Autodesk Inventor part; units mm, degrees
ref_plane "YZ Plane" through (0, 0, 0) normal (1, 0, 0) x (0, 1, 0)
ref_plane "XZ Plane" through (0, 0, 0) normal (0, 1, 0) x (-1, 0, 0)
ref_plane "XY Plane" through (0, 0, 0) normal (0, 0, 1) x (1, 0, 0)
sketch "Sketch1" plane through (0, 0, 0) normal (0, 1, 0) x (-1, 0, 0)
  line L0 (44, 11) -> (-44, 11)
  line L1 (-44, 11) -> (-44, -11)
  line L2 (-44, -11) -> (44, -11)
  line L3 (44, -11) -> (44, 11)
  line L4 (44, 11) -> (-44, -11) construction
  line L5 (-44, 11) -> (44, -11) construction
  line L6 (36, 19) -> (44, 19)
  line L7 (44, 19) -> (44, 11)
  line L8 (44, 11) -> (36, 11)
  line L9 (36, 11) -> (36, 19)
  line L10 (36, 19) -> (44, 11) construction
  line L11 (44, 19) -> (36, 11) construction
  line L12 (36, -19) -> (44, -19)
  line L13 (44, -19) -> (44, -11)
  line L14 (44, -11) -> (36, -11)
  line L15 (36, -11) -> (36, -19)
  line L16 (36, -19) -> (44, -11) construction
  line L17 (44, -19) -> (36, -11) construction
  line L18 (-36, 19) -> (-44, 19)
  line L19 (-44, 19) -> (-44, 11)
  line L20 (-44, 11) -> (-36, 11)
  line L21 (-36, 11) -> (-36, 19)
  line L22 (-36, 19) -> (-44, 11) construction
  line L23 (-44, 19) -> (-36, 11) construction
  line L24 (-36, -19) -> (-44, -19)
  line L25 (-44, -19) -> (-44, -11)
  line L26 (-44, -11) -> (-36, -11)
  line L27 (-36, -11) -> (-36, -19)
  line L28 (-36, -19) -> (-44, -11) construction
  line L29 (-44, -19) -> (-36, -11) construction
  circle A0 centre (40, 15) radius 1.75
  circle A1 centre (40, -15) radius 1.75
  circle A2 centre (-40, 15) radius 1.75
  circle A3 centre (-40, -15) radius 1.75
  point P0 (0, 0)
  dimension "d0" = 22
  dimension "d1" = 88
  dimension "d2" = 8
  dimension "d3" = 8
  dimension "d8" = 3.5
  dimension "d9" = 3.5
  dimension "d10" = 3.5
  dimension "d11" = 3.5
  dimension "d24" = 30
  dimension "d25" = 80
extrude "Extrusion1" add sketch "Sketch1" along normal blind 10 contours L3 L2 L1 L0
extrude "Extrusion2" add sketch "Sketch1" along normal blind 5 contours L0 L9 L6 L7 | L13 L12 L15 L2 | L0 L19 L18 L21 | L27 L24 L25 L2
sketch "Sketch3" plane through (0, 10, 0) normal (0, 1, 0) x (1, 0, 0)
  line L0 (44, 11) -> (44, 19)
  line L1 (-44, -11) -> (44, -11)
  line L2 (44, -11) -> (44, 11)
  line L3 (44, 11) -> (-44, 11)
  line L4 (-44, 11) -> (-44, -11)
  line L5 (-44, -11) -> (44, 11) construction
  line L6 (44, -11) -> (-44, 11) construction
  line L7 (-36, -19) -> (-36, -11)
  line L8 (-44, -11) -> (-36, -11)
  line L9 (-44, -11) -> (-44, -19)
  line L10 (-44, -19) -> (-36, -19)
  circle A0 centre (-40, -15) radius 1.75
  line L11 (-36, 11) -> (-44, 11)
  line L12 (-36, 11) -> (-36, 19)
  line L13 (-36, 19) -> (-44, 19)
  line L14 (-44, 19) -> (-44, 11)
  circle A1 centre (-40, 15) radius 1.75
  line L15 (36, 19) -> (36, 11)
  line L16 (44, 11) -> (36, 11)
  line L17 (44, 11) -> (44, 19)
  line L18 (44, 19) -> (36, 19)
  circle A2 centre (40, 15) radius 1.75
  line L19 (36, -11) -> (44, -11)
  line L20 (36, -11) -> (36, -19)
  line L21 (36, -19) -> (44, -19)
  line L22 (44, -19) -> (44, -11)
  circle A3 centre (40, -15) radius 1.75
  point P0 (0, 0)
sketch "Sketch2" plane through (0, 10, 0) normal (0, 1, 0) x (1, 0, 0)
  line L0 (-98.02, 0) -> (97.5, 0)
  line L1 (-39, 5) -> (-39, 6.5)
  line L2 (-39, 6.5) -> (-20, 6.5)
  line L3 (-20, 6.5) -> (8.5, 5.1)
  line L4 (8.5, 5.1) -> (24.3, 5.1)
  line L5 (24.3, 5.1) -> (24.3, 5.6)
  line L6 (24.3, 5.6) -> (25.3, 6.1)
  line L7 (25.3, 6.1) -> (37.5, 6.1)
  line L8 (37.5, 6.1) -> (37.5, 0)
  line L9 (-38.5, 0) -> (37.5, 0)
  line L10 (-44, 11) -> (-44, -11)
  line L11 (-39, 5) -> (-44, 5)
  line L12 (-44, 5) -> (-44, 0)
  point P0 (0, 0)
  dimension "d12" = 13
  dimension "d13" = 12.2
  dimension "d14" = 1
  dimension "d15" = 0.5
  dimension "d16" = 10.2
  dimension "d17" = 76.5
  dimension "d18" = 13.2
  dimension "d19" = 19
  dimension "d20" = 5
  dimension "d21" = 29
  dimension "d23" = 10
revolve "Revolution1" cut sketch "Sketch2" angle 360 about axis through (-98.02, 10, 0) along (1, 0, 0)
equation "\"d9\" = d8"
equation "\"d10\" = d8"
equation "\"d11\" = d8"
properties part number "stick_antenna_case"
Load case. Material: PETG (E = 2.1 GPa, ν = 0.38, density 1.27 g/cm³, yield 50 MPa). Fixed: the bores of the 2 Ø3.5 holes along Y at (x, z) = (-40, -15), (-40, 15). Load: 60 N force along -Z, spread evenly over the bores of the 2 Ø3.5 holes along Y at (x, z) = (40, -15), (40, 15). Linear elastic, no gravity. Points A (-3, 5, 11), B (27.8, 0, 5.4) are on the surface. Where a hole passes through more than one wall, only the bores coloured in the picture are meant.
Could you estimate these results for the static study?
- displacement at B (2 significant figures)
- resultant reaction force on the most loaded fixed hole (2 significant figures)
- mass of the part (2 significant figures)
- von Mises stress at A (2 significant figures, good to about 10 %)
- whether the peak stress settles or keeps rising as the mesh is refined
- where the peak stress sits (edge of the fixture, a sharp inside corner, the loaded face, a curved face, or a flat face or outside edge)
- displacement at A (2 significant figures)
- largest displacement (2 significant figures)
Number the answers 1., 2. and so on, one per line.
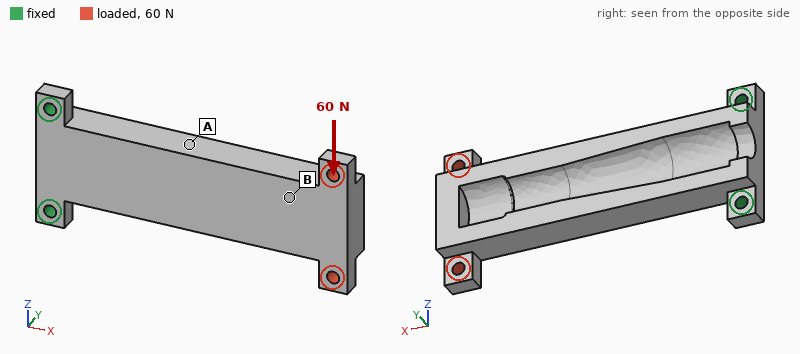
1. 0.74 mm
2. 190 N
3. 20 g
4. 3.3 MPa
5. keeps rising
6. edge of the fixture
7. 0.32 mm
8. 1.0 mm
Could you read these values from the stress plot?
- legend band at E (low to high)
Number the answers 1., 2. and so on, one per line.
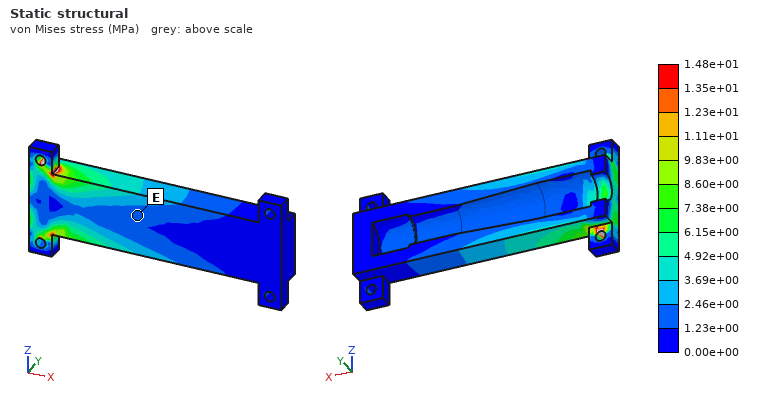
1. 1.23e+00 to 2.46e+00 MPa
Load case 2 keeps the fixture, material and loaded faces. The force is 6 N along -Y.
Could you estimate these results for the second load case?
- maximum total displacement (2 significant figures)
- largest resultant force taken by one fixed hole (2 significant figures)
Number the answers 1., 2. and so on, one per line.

1. 0.98 mm
2. 7.2 N
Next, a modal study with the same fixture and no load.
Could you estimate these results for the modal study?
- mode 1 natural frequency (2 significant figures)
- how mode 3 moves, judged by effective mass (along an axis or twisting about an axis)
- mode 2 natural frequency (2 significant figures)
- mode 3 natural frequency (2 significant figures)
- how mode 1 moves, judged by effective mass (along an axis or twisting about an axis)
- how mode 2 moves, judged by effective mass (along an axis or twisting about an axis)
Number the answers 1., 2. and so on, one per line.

1. 150 Hz
2. twisting about X
3. 490 Hz
4. 850 Hz
5. along Y
6. along Z
